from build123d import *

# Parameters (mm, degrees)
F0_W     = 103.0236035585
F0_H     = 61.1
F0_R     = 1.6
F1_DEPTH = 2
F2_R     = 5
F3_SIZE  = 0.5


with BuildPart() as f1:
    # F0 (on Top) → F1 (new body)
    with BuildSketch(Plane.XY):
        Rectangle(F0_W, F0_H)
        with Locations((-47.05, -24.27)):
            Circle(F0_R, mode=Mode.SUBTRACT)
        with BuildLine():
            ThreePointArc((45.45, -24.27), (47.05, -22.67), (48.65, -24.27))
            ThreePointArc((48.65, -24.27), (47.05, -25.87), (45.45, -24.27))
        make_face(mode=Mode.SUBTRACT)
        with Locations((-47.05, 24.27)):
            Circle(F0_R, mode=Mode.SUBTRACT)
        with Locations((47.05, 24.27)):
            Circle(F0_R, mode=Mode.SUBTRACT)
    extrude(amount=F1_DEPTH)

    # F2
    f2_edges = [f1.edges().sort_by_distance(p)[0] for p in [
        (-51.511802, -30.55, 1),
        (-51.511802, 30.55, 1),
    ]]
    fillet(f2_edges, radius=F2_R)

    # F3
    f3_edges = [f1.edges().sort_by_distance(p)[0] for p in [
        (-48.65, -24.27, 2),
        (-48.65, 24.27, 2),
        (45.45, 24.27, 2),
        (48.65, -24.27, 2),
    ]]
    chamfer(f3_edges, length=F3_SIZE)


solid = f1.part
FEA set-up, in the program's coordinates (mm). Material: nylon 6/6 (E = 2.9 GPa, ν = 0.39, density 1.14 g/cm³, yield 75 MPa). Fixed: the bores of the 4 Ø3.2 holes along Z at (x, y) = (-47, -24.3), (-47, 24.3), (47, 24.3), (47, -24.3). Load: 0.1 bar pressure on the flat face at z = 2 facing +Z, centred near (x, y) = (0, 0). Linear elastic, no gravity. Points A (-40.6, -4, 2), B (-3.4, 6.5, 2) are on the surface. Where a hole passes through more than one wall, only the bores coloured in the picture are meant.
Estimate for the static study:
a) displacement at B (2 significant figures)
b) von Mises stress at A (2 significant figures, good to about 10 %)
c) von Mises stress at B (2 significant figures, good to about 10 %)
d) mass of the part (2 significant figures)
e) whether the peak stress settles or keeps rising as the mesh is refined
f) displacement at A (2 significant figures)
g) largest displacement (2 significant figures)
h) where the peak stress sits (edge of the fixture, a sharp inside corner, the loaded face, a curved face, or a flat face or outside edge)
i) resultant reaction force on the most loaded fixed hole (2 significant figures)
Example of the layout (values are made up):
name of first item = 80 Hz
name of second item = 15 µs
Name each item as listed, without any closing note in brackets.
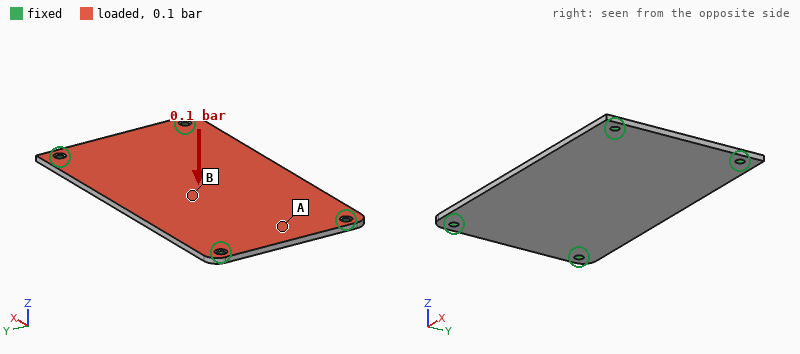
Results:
displacement at B = 1.4 mm
von Mises stress at A = 2.7 MPa
von Mises stress at B = 5.7 MPa
mass of the part = 14 g
whether the peak stress settles or keeps rising as the mesh is refined = keeps rising
displacement at A = 0.29 mm
largest displacement = 1.4 mm
where the peak stress sits = edge of the fixture
resultant reaction force on the most loaded fixed hole = 16 N
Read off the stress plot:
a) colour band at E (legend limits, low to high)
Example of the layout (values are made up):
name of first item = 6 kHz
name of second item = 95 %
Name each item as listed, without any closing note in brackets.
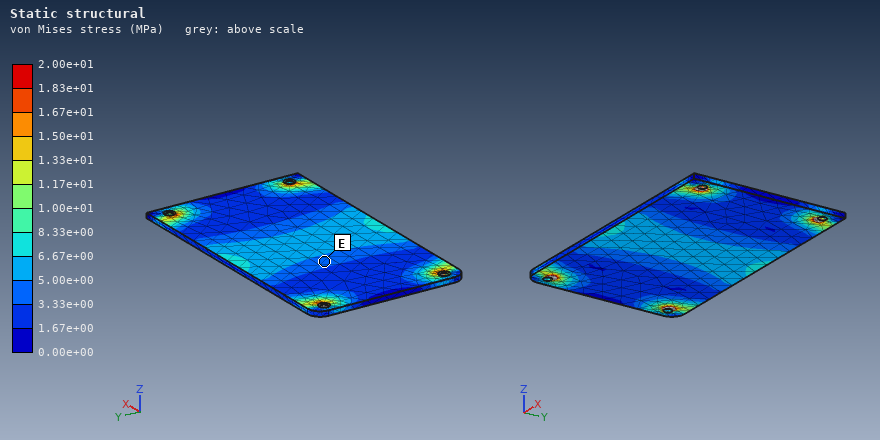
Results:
colour band at E = 3.33e+00 to 5.00e+00 MPa
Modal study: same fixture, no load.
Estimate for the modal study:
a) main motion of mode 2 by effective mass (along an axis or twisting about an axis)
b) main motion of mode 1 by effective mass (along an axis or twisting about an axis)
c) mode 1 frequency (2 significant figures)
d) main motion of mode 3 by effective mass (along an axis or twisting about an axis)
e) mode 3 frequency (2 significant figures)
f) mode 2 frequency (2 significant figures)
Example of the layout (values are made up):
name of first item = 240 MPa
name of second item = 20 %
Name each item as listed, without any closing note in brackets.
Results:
main motion of mode 2 by effective mass = twisting about X
main motion of mode 1 by effective mass = along Z
mode 1 frequency = 320 Hz
main motion of mode 3 by effective mass = twisting about Y
mode 3 frequency = 890 Hz
mode 2 frequency = 520 Hz
